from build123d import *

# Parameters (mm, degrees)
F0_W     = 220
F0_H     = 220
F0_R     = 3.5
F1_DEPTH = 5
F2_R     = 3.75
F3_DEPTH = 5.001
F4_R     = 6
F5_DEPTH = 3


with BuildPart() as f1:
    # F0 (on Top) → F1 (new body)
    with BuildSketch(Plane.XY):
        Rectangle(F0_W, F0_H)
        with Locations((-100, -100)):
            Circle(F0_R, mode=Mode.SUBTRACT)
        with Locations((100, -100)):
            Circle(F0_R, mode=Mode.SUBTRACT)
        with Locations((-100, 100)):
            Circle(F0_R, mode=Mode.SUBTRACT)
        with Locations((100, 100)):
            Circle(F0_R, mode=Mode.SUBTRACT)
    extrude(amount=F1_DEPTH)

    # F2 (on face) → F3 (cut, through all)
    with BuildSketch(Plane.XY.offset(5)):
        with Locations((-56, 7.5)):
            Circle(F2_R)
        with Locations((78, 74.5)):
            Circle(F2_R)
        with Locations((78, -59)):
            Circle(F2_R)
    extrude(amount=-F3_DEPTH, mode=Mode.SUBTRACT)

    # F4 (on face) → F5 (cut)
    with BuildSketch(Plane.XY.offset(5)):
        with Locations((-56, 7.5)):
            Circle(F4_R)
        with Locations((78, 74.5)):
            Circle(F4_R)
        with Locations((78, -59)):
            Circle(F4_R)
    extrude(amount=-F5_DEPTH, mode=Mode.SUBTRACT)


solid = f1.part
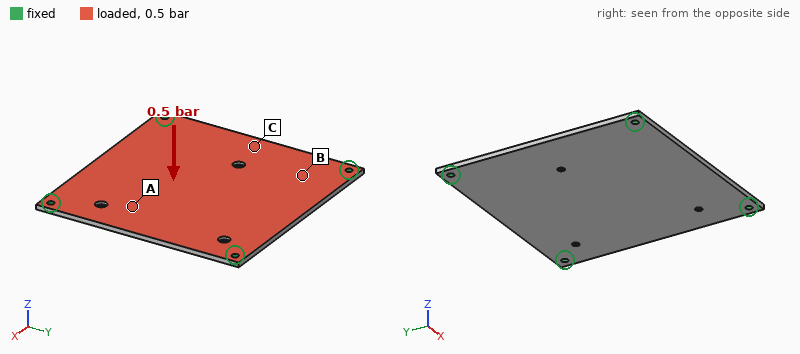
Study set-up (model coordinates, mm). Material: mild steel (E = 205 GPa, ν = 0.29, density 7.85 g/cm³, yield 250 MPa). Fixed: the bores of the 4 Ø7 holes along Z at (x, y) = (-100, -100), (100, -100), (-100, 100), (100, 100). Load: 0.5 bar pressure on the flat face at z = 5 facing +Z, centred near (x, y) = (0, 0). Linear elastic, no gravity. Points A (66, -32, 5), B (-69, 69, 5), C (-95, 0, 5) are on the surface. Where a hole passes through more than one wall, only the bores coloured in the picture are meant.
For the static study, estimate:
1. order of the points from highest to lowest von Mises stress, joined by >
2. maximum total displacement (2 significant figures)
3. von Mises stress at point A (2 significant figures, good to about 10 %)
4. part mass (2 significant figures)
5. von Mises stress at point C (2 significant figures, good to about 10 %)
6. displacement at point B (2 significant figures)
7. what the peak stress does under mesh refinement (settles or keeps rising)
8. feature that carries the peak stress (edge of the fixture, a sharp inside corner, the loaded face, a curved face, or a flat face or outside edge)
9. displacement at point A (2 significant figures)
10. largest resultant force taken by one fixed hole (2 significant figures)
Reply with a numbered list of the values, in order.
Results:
1. C > A > B
2. 0.31 mm
3. 22 MPa
4. 1.9 kg
5. 31 MPa
6. 0.12 mm
7. keeps rising
8. edge of the fixture
9. 0.20 mm
10. 600 N
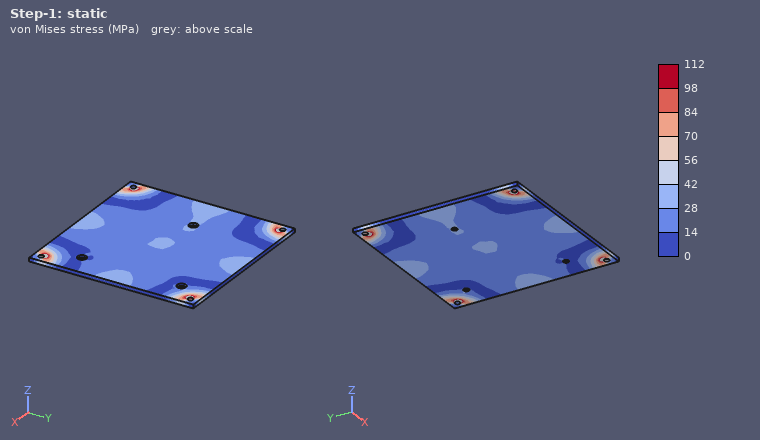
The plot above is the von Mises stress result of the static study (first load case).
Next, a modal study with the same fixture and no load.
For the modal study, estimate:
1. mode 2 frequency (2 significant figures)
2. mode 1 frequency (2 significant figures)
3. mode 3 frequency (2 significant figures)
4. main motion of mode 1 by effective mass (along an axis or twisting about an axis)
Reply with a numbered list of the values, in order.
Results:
1. 710 Hz
2. 390 Hz
3. 710 Hz
4. along Z
